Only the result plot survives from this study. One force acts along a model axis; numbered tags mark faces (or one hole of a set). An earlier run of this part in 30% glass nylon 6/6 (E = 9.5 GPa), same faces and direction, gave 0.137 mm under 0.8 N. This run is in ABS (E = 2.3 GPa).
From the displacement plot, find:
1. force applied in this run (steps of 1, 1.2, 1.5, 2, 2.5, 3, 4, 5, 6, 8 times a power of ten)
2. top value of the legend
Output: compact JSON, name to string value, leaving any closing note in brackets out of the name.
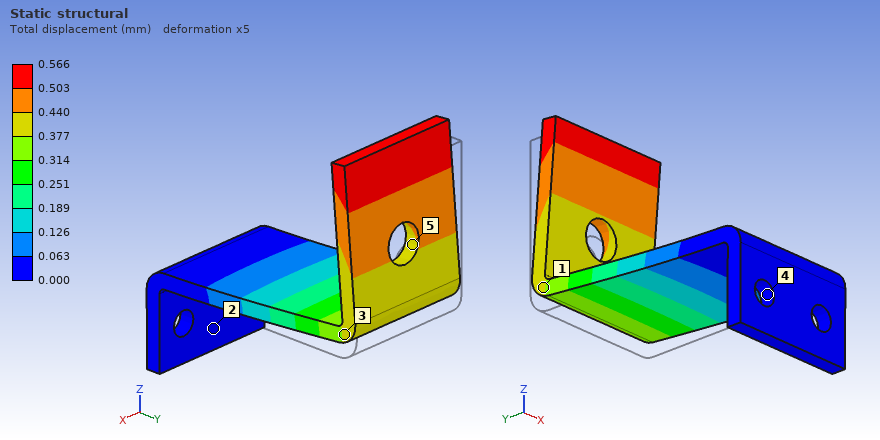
{"force applied in this run": "0.8 N", "top value of the legend": "0.566 mm"}
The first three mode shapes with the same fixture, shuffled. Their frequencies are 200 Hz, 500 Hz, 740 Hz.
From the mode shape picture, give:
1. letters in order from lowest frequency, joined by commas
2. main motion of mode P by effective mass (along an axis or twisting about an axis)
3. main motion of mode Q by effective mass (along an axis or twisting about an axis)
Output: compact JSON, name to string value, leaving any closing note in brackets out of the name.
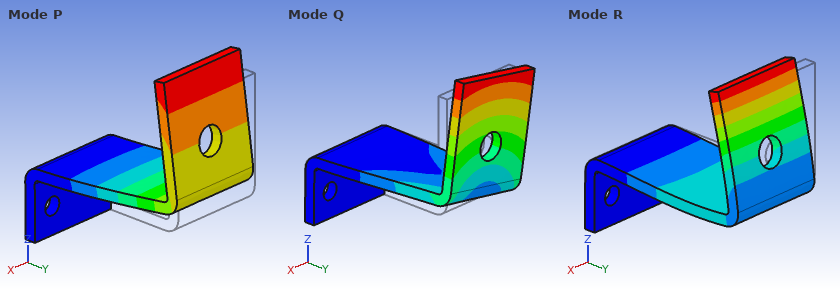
{"letters in order from lowest frequency, joined by commas": "P, Q, R", "main motion of mode P by effective mass": "along Z", "main motion of mode Q by effective mass": "along X"}
